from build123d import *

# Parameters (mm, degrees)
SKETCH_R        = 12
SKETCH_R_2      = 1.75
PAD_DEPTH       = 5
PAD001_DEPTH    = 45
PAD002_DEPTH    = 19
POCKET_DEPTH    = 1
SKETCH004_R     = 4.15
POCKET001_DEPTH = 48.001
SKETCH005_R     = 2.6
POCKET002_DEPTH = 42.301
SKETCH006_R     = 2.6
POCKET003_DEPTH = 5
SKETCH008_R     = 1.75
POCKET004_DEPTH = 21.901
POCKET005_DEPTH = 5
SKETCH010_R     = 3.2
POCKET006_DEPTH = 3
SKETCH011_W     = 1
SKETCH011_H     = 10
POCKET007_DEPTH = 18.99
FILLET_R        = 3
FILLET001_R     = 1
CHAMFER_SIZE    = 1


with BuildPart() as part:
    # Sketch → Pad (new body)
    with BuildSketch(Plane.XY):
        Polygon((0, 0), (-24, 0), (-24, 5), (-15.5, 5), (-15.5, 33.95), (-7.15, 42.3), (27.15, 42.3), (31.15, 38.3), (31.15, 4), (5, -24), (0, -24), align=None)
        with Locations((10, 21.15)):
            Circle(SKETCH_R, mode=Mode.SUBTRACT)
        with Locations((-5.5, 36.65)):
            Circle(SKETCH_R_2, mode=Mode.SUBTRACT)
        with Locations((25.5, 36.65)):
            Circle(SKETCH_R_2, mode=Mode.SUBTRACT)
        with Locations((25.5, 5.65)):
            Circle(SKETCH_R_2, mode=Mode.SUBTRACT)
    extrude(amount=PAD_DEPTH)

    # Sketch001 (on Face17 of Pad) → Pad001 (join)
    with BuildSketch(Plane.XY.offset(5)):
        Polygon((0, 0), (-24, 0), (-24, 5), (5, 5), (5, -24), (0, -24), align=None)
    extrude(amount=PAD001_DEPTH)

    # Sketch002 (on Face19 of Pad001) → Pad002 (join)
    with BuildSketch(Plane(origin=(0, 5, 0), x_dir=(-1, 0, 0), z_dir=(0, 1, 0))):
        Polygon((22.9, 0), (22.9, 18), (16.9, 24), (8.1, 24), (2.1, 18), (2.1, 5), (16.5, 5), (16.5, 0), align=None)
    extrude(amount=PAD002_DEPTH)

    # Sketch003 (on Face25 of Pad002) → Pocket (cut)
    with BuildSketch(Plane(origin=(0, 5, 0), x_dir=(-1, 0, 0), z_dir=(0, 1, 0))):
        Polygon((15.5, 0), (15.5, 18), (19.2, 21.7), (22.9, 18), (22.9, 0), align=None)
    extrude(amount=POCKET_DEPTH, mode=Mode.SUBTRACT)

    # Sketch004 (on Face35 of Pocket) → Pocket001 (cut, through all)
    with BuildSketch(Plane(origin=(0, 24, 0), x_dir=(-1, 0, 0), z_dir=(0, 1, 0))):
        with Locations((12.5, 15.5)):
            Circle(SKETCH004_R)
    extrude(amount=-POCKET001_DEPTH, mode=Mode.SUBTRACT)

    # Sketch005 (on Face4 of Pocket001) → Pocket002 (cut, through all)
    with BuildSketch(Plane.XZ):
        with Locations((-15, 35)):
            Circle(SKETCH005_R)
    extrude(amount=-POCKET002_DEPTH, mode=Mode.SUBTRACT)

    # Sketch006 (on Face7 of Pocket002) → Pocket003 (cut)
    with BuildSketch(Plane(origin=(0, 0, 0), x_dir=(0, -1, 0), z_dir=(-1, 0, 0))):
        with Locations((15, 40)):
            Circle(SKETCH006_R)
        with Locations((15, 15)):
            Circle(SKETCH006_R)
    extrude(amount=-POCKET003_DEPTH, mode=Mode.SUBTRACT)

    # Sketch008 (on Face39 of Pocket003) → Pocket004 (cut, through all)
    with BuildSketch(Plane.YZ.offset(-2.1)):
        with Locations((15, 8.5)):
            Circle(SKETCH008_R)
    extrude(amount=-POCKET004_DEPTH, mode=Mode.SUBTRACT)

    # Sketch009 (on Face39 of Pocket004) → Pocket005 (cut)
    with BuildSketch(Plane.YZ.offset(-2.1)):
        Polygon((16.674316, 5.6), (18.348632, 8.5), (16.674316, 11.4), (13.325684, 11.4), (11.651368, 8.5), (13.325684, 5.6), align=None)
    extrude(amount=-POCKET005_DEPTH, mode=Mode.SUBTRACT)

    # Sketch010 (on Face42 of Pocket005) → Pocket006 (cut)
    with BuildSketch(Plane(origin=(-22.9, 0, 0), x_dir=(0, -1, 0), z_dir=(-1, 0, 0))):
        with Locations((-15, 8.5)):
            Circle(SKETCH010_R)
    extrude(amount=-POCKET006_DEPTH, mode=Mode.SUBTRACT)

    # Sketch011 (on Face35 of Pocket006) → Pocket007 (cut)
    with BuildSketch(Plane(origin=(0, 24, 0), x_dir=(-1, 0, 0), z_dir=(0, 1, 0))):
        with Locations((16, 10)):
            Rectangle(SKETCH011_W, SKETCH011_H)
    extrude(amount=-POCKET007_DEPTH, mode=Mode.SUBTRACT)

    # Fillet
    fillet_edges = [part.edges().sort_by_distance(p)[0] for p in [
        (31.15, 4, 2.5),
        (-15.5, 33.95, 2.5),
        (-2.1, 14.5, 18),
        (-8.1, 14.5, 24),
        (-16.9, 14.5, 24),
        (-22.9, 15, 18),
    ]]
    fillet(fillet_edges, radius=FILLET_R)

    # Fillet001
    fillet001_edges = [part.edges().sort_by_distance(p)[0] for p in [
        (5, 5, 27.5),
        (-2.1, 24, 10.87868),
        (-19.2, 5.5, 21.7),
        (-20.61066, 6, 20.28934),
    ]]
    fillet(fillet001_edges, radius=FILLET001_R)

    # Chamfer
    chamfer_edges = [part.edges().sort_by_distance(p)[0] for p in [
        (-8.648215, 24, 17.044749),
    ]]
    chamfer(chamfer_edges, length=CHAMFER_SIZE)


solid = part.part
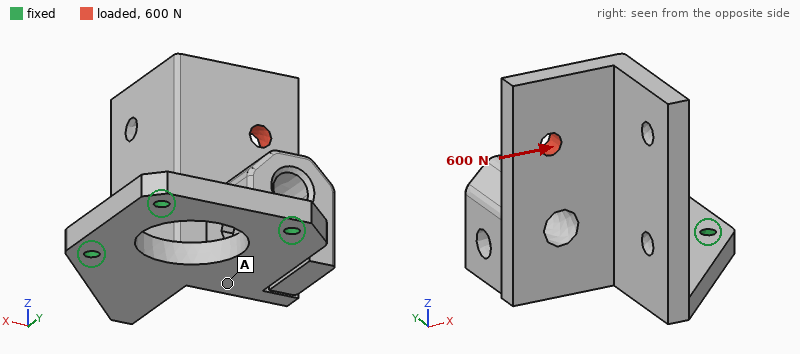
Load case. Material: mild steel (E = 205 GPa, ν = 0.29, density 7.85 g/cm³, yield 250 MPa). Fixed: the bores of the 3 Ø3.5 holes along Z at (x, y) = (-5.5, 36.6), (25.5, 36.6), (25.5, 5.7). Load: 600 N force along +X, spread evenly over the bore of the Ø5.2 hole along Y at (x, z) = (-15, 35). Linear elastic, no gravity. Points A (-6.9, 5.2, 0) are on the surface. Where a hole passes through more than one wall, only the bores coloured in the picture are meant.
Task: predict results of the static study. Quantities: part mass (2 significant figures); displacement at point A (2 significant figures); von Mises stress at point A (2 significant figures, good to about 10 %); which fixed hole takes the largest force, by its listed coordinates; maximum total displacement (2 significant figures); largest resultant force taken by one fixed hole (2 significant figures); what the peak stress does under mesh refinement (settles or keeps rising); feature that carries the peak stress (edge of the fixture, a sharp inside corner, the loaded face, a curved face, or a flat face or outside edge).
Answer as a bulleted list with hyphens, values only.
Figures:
- 210 g
- 0.051 mm
- 19 MPa
- (25.5, 5.7)
- 0.21 mm
- 560 N
- keeps rising
- edge of the fixture
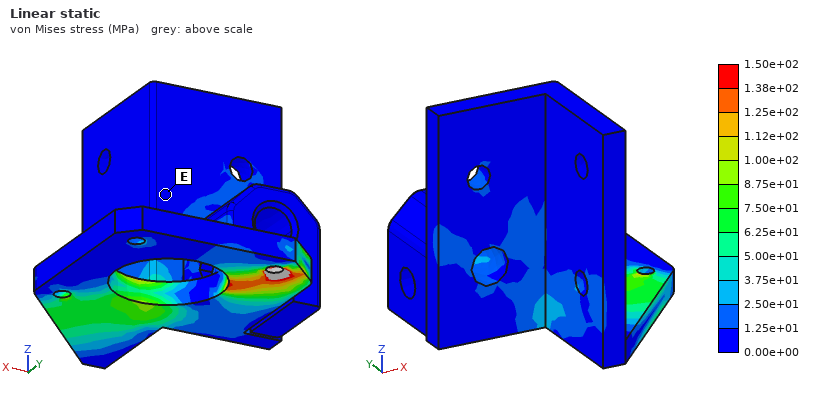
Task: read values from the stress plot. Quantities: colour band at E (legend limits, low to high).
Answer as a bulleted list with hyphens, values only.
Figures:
- 0.00e+00 to 1.25e+01 MPa
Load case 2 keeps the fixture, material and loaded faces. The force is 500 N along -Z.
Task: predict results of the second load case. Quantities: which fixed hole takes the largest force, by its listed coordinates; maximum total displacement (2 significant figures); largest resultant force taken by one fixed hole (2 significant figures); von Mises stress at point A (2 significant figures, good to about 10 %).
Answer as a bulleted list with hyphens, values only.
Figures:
- (-5.5, 36.6)
- 0.16 mm
- 350 N
- 12 MPa
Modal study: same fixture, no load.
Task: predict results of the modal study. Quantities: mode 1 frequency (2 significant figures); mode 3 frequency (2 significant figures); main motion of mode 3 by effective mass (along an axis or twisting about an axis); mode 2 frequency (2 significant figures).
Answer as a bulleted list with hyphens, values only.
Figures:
- 890 Hz
- 4100 Hz
- along Z
- 2200 Hz
